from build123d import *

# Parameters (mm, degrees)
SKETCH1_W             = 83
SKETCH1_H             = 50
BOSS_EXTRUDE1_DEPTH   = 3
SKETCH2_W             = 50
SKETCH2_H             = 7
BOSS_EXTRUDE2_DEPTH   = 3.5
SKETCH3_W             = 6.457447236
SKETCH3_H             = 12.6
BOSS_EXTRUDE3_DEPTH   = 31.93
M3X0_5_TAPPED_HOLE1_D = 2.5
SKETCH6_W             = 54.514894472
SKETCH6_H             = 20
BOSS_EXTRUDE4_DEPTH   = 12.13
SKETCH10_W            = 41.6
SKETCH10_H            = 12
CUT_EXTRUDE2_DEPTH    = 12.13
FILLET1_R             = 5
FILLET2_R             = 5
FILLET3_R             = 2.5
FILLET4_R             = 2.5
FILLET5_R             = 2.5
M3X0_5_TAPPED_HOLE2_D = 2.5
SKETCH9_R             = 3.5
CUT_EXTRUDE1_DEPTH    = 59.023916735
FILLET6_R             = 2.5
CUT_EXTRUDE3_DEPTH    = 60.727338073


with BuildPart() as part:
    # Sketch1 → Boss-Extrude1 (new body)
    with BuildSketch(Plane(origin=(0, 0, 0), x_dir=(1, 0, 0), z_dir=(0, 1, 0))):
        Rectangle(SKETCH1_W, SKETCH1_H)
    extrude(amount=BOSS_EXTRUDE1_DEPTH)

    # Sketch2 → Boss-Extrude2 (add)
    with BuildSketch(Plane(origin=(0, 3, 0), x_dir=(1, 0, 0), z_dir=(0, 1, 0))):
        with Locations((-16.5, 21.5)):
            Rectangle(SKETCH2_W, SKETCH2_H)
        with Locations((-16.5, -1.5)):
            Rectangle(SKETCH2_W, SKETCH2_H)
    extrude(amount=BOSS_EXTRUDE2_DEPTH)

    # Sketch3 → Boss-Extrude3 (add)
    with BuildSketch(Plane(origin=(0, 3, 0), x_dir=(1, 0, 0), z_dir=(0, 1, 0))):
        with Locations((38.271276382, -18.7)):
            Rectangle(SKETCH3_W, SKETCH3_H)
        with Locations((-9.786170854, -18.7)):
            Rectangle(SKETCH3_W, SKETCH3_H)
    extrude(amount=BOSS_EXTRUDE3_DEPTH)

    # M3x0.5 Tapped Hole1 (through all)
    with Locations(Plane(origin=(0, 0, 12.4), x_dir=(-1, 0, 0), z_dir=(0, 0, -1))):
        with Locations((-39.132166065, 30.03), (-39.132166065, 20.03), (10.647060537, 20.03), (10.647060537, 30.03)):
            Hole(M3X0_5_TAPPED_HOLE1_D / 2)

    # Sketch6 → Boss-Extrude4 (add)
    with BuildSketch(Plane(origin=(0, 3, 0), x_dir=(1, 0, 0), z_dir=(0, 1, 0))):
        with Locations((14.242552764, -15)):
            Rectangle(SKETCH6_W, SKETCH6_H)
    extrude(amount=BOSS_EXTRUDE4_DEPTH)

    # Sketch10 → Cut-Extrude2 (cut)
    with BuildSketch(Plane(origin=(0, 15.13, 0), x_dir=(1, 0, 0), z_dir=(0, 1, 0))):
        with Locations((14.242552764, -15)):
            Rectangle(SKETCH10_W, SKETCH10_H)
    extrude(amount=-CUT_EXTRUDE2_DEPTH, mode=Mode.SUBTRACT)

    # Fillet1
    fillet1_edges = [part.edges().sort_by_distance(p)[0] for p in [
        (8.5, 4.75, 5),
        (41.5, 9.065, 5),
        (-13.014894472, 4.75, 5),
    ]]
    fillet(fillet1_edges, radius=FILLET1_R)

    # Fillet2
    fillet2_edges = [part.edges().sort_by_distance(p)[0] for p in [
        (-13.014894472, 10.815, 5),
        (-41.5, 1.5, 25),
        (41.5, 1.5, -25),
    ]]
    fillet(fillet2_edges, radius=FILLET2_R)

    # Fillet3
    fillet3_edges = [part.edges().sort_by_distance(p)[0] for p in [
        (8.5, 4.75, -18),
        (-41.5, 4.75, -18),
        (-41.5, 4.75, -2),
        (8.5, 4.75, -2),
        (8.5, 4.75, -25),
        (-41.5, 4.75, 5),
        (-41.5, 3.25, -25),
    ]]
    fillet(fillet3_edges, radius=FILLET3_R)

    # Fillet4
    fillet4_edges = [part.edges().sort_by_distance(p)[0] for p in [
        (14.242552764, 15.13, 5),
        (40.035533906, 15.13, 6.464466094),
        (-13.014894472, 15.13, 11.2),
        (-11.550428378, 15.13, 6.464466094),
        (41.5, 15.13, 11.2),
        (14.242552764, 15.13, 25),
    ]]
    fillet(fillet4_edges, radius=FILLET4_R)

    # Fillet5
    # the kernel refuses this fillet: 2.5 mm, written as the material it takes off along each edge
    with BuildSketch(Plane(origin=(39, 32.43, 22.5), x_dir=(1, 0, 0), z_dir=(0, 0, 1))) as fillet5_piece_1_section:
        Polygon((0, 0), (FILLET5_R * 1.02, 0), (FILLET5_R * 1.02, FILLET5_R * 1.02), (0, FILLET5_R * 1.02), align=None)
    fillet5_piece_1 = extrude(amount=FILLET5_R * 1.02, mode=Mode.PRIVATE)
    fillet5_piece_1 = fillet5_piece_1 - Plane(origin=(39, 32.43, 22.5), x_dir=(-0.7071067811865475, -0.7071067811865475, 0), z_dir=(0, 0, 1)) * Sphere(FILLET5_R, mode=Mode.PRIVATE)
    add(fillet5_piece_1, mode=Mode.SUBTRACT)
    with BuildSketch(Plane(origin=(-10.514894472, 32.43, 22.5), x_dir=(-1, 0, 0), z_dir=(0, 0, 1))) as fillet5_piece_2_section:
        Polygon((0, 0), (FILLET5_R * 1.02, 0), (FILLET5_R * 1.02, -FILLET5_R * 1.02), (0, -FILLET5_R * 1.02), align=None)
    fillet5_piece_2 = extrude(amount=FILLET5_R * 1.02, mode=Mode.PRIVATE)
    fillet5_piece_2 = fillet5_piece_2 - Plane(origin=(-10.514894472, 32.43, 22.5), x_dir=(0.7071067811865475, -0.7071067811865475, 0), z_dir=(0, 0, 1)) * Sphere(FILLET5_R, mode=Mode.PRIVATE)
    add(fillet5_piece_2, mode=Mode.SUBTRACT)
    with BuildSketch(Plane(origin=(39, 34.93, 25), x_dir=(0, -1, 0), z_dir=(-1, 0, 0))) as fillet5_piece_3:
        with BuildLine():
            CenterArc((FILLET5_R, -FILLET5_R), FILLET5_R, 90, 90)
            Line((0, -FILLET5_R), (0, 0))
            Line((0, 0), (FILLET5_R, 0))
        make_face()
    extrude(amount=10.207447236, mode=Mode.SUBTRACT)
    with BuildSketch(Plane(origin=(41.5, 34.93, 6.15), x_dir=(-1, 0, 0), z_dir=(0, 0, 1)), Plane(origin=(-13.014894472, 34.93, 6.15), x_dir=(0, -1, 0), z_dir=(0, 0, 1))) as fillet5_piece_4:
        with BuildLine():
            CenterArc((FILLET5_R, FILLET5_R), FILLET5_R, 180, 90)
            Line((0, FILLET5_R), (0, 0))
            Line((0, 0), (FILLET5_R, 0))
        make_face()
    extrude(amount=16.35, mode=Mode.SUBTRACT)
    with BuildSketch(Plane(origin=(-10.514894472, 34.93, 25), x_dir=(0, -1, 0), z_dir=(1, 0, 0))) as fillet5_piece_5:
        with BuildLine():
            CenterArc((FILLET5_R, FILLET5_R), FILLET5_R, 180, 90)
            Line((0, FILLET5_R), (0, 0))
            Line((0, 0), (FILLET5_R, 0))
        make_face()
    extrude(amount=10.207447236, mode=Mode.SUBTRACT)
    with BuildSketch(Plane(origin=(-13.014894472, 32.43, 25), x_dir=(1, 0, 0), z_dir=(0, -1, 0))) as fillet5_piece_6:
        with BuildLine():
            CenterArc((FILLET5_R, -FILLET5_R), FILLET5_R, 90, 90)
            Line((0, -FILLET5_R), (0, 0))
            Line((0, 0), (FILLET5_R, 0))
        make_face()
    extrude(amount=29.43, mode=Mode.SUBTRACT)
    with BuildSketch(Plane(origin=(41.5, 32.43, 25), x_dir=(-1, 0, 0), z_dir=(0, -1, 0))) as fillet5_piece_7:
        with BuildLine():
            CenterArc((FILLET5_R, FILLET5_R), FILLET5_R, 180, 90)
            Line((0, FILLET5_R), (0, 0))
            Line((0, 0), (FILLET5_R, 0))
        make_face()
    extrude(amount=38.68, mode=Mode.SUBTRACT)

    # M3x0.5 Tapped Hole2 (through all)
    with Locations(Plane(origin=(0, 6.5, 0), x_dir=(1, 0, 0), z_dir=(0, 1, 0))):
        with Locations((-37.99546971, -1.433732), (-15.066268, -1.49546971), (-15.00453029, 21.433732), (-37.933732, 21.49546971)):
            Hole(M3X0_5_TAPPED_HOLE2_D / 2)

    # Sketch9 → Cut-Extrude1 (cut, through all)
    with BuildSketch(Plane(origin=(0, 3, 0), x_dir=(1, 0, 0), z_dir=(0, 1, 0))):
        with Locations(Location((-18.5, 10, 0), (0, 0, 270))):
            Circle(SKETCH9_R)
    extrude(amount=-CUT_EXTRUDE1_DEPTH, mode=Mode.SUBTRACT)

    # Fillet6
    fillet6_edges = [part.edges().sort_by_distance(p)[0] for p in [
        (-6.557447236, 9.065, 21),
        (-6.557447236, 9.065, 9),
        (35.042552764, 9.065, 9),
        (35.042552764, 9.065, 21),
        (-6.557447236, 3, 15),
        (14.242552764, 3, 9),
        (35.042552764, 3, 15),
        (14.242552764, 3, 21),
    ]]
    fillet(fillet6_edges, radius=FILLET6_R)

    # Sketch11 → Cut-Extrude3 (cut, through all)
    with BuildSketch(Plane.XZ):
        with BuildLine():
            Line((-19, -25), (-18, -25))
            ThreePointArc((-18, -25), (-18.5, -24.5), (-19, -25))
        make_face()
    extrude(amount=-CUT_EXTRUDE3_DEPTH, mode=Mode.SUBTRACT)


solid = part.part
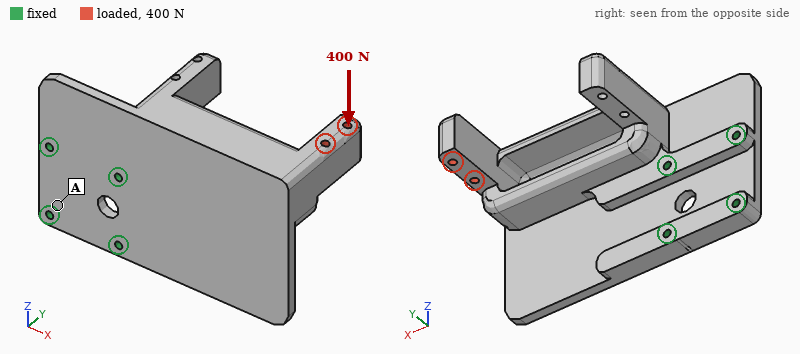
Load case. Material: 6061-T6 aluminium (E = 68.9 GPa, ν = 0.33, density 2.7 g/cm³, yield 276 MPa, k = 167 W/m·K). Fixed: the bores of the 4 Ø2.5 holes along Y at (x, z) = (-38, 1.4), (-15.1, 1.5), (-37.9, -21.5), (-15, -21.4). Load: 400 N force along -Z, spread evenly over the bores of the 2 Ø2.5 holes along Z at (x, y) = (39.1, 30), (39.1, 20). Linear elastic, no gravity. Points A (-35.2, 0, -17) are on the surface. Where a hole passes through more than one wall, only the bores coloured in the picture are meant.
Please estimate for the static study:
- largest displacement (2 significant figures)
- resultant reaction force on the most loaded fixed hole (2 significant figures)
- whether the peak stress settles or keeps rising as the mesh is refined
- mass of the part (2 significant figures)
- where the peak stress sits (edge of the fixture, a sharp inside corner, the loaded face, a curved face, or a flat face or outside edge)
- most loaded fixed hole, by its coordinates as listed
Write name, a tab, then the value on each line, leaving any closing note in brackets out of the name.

largest displacement	0.38 mm
resultant reaction force on the most loaded fixed hole	780 N
whether the peak stress settles or keeps rising as the mesh is refined	keeps rising
mass of the part	66 g
where the peak stress sits	edge of the fixture
most loaded fixed hole, by its coordinates as listed	(-15.1, 1.5)
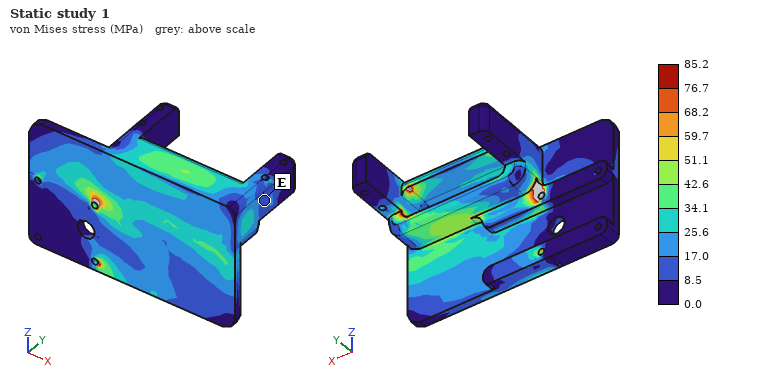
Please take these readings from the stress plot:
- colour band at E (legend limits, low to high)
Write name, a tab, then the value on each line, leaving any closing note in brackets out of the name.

colour band at E	8.5 to 17.0 MPa
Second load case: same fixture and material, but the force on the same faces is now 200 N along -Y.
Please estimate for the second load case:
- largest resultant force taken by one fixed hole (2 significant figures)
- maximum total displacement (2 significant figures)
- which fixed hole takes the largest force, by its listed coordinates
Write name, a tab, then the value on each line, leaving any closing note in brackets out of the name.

largest resultant force taken by one fixed hole	730 N
maximum total displacement	0.32 mm
which fixed hole takes the largest force, by its listed coordinates	(-15.1, 1.5)
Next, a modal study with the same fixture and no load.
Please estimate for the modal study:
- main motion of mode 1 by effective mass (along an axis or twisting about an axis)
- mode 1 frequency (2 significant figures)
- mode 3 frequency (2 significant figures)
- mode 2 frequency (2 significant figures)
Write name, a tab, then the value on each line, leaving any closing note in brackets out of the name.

main motion of mode 1 by effective mass	along Y
mode 1 frequency	1100 Hz
mode 3 frequency	4100 Hz
mode 2 frequency	2100 Hz
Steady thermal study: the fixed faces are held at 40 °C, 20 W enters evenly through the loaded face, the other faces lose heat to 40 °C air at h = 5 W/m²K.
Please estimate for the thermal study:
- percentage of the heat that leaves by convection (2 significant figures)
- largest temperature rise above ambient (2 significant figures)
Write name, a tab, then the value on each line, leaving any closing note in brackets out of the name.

percentage of the heat that leaves by convection	4.9 %
largest temperature rise above ambient	57 K
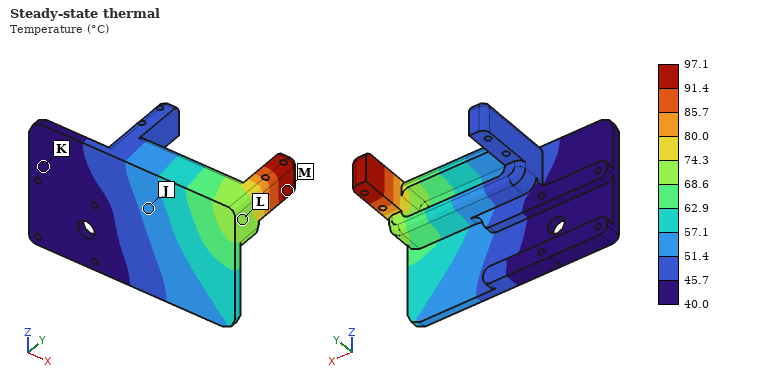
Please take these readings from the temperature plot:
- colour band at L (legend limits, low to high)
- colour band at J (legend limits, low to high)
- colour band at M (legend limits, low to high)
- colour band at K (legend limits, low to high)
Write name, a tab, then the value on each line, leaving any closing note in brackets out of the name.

colour band at L	68.6 to 74.3 °C
colour band at J	51.4 to 57.1 °C
colour band at M	91.4 to 97.1 °C
colour band at K	40.0 to 45.7 °C
